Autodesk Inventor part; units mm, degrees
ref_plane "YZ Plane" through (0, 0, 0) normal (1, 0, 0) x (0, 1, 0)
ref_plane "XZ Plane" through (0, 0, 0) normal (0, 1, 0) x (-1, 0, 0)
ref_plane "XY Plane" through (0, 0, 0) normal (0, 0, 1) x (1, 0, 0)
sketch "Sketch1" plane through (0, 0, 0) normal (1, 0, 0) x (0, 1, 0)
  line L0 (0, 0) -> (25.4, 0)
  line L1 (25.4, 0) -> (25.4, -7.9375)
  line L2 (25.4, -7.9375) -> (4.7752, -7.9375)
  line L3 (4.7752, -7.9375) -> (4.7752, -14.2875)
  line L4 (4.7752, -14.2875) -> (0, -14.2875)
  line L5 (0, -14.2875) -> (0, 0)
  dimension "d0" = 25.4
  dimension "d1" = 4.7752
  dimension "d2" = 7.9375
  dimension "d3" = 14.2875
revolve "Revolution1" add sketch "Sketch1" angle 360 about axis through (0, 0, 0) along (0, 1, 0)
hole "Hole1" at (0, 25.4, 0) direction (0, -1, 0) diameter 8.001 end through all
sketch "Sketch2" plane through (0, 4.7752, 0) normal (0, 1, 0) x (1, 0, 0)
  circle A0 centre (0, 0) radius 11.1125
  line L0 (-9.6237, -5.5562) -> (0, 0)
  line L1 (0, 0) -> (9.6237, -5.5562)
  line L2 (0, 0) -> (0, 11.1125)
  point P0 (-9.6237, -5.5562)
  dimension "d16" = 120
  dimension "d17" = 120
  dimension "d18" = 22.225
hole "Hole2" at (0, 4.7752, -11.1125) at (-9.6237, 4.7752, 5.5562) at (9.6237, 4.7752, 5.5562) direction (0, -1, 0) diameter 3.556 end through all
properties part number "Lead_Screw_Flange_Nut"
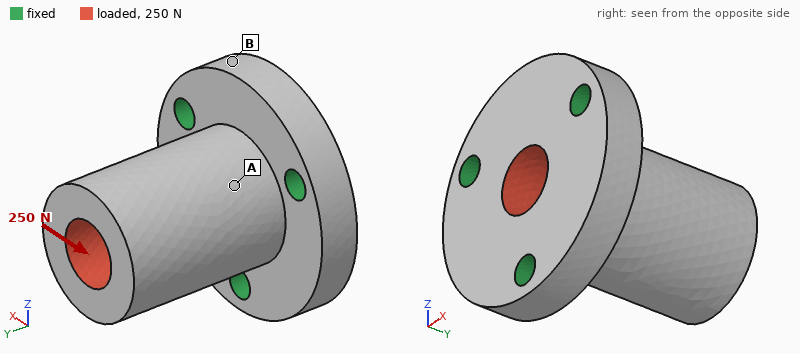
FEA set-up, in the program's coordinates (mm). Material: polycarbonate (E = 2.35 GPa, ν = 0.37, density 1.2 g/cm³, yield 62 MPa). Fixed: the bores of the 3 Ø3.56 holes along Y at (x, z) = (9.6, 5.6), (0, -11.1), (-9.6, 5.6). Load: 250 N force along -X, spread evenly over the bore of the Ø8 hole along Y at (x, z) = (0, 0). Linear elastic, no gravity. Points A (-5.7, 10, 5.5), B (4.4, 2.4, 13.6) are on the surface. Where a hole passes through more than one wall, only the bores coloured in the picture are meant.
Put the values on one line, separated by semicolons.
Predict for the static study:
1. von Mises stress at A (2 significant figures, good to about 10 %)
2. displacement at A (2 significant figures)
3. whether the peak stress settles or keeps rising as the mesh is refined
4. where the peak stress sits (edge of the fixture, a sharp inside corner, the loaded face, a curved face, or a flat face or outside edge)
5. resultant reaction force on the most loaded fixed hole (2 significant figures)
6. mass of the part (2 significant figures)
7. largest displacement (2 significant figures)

3.1 MPa; 0.042 mm; keeps rising; edge of the fixture; 160 N; 6.9 g; 0.13 mm
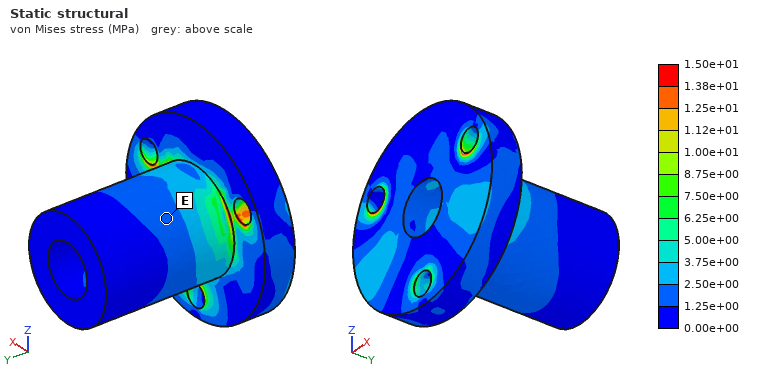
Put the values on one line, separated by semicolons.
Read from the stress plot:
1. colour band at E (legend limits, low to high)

1.25e+00 to 2.50e+00 MPa
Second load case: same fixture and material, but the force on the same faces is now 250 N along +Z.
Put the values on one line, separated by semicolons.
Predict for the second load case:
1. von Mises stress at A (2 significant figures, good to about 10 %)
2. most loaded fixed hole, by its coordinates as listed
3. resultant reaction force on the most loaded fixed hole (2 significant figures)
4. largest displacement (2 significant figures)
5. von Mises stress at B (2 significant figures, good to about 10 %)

2.4 MPa; (0, -11.1); 180 N; 0.13 mm; 1.8 MPa
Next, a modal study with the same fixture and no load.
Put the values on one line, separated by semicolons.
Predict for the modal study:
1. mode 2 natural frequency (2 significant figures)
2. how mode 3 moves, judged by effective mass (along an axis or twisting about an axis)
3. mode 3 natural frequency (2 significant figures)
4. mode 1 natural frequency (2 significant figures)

3900 Hz; along Y; 8900 Hz; 3900 Hz
